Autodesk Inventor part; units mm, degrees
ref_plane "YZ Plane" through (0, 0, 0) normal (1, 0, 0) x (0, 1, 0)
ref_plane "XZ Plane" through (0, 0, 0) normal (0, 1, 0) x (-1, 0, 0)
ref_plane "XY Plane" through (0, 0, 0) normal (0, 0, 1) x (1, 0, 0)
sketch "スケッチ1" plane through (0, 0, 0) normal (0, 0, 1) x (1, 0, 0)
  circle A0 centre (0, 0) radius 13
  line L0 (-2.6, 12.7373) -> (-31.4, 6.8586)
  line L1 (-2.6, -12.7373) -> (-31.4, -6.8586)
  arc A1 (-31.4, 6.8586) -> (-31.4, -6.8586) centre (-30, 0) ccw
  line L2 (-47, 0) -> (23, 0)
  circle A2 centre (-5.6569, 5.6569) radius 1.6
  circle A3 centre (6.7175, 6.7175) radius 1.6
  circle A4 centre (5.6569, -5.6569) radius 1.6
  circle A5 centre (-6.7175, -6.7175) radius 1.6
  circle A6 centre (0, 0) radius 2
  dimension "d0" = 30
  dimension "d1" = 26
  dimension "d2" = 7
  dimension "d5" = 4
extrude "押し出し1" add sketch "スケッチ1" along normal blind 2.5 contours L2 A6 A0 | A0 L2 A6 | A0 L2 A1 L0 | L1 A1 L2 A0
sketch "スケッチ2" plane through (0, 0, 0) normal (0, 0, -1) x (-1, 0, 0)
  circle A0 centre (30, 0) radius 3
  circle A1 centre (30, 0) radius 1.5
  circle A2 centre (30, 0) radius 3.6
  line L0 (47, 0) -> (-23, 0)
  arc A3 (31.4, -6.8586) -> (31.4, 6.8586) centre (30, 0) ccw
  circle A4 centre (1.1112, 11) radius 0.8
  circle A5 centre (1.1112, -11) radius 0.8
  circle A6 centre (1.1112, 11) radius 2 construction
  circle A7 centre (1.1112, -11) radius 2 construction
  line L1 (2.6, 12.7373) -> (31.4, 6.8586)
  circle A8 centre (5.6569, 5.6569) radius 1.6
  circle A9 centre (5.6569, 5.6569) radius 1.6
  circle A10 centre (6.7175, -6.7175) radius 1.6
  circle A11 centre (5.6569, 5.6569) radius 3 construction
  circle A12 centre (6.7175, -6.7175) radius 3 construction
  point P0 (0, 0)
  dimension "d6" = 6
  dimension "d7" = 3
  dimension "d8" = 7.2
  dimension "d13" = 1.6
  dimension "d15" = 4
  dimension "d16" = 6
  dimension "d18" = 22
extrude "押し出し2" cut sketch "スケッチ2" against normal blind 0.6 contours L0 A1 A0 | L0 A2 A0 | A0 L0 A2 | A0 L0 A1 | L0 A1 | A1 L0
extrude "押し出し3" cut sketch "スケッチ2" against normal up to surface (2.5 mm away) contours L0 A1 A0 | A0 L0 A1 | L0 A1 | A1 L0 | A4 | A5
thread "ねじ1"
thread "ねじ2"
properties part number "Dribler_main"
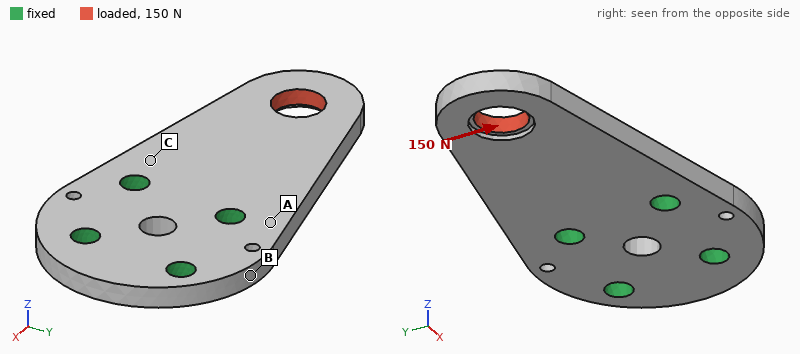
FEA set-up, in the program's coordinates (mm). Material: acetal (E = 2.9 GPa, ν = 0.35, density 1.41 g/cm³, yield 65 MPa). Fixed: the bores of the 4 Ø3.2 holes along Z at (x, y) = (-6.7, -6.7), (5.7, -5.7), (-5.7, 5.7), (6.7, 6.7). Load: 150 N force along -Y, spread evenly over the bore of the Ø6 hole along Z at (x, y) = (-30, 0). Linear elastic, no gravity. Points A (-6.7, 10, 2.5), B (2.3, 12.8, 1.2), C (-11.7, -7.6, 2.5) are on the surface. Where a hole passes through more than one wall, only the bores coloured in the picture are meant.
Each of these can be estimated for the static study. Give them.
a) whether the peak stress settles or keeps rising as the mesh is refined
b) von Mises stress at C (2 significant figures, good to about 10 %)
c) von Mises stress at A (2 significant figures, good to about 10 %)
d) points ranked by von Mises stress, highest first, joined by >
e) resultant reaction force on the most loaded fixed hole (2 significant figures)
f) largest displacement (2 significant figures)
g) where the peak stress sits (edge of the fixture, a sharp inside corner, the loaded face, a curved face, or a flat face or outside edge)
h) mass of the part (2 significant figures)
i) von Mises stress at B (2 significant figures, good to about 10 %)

keeps rising
11 MPa
7.0 MPa
C > A > B
230 N
0.30 mm
edge of the fixture
3.1 g
2.6 MPa
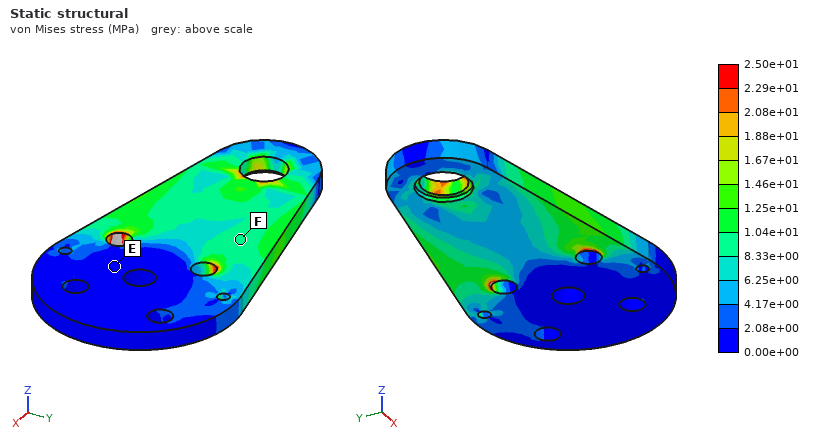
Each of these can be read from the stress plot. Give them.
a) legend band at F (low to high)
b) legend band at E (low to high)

8.33e+00 to 1.04e+01 MPa
0.00e+00 to 2.08e+00 MPa
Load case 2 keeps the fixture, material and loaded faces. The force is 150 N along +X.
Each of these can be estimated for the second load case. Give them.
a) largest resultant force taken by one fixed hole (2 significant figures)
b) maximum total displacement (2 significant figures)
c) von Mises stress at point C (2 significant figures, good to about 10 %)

71 N
0.27 mm
5.1 MPa
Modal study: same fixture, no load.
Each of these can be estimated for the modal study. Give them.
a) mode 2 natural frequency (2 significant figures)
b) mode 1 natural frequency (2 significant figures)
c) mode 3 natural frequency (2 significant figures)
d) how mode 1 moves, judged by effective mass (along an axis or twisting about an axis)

3200 Hz
910 Hz
4200 Hz
along Z
